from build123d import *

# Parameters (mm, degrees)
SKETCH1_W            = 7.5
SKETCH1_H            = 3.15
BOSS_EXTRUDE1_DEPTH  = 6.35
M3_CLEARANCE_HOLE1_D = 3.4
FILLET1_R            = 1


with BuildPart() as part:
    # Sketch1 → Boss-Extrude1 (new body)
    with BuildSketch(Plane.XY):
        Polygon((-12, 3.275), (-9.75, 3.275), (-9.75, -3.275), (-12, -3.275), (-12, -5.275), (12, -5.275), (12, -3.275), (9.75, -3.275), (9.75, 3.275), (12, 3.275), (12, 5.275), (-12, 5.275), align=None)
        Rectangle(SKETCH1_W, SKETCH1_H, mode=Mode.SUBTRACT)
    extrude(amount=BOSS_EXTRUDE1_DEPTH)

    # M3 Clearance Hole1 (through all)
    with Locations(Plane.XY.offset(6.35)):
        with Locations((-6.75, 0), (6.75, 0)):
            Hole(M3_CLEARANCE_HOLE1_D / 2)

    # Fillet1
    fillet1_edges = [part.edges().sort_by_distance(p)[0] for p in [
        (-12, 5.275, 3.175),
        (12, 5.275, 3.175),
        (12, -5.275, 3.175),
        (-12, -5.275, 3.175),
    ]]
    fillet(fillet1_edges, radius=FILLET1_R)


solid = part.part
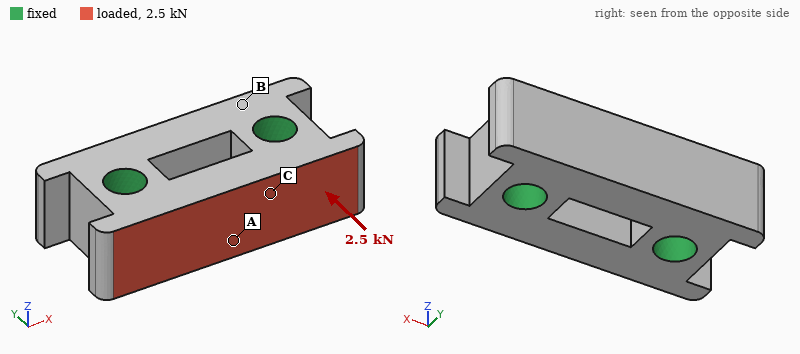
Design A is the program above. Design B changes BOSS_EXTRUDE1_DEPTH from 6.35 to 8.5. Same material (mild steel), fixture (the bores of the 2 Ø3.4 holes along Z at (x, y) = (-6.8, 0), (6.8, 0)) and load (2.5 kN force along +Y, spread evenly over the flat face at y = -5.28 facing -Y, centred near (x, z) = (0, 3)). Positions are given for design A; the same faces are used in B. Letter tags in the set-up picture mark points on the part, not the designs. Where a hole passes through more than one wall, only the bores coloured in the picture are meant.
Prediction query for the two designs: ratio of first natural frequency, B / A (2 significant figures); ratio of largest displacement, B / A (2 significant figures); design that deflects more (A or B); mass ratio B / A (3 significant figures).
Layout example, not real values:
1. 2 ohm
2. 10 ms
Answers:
1. 1.0
2. 0.76
3. A
4. 1.34
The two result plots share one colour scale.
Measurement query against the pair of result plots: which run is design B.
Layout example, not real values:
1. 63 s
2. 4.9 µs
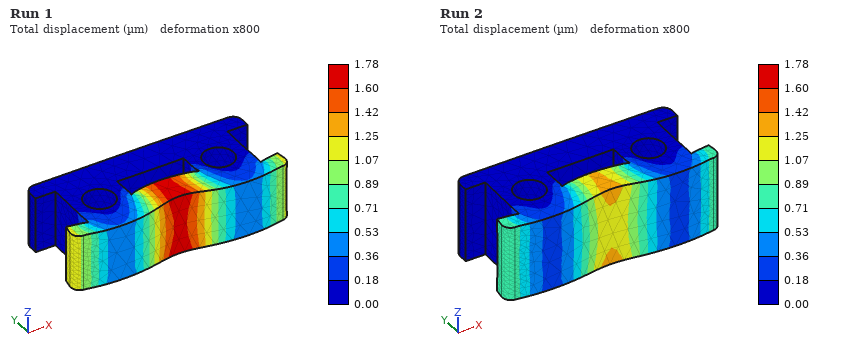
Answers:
1. Run 2
